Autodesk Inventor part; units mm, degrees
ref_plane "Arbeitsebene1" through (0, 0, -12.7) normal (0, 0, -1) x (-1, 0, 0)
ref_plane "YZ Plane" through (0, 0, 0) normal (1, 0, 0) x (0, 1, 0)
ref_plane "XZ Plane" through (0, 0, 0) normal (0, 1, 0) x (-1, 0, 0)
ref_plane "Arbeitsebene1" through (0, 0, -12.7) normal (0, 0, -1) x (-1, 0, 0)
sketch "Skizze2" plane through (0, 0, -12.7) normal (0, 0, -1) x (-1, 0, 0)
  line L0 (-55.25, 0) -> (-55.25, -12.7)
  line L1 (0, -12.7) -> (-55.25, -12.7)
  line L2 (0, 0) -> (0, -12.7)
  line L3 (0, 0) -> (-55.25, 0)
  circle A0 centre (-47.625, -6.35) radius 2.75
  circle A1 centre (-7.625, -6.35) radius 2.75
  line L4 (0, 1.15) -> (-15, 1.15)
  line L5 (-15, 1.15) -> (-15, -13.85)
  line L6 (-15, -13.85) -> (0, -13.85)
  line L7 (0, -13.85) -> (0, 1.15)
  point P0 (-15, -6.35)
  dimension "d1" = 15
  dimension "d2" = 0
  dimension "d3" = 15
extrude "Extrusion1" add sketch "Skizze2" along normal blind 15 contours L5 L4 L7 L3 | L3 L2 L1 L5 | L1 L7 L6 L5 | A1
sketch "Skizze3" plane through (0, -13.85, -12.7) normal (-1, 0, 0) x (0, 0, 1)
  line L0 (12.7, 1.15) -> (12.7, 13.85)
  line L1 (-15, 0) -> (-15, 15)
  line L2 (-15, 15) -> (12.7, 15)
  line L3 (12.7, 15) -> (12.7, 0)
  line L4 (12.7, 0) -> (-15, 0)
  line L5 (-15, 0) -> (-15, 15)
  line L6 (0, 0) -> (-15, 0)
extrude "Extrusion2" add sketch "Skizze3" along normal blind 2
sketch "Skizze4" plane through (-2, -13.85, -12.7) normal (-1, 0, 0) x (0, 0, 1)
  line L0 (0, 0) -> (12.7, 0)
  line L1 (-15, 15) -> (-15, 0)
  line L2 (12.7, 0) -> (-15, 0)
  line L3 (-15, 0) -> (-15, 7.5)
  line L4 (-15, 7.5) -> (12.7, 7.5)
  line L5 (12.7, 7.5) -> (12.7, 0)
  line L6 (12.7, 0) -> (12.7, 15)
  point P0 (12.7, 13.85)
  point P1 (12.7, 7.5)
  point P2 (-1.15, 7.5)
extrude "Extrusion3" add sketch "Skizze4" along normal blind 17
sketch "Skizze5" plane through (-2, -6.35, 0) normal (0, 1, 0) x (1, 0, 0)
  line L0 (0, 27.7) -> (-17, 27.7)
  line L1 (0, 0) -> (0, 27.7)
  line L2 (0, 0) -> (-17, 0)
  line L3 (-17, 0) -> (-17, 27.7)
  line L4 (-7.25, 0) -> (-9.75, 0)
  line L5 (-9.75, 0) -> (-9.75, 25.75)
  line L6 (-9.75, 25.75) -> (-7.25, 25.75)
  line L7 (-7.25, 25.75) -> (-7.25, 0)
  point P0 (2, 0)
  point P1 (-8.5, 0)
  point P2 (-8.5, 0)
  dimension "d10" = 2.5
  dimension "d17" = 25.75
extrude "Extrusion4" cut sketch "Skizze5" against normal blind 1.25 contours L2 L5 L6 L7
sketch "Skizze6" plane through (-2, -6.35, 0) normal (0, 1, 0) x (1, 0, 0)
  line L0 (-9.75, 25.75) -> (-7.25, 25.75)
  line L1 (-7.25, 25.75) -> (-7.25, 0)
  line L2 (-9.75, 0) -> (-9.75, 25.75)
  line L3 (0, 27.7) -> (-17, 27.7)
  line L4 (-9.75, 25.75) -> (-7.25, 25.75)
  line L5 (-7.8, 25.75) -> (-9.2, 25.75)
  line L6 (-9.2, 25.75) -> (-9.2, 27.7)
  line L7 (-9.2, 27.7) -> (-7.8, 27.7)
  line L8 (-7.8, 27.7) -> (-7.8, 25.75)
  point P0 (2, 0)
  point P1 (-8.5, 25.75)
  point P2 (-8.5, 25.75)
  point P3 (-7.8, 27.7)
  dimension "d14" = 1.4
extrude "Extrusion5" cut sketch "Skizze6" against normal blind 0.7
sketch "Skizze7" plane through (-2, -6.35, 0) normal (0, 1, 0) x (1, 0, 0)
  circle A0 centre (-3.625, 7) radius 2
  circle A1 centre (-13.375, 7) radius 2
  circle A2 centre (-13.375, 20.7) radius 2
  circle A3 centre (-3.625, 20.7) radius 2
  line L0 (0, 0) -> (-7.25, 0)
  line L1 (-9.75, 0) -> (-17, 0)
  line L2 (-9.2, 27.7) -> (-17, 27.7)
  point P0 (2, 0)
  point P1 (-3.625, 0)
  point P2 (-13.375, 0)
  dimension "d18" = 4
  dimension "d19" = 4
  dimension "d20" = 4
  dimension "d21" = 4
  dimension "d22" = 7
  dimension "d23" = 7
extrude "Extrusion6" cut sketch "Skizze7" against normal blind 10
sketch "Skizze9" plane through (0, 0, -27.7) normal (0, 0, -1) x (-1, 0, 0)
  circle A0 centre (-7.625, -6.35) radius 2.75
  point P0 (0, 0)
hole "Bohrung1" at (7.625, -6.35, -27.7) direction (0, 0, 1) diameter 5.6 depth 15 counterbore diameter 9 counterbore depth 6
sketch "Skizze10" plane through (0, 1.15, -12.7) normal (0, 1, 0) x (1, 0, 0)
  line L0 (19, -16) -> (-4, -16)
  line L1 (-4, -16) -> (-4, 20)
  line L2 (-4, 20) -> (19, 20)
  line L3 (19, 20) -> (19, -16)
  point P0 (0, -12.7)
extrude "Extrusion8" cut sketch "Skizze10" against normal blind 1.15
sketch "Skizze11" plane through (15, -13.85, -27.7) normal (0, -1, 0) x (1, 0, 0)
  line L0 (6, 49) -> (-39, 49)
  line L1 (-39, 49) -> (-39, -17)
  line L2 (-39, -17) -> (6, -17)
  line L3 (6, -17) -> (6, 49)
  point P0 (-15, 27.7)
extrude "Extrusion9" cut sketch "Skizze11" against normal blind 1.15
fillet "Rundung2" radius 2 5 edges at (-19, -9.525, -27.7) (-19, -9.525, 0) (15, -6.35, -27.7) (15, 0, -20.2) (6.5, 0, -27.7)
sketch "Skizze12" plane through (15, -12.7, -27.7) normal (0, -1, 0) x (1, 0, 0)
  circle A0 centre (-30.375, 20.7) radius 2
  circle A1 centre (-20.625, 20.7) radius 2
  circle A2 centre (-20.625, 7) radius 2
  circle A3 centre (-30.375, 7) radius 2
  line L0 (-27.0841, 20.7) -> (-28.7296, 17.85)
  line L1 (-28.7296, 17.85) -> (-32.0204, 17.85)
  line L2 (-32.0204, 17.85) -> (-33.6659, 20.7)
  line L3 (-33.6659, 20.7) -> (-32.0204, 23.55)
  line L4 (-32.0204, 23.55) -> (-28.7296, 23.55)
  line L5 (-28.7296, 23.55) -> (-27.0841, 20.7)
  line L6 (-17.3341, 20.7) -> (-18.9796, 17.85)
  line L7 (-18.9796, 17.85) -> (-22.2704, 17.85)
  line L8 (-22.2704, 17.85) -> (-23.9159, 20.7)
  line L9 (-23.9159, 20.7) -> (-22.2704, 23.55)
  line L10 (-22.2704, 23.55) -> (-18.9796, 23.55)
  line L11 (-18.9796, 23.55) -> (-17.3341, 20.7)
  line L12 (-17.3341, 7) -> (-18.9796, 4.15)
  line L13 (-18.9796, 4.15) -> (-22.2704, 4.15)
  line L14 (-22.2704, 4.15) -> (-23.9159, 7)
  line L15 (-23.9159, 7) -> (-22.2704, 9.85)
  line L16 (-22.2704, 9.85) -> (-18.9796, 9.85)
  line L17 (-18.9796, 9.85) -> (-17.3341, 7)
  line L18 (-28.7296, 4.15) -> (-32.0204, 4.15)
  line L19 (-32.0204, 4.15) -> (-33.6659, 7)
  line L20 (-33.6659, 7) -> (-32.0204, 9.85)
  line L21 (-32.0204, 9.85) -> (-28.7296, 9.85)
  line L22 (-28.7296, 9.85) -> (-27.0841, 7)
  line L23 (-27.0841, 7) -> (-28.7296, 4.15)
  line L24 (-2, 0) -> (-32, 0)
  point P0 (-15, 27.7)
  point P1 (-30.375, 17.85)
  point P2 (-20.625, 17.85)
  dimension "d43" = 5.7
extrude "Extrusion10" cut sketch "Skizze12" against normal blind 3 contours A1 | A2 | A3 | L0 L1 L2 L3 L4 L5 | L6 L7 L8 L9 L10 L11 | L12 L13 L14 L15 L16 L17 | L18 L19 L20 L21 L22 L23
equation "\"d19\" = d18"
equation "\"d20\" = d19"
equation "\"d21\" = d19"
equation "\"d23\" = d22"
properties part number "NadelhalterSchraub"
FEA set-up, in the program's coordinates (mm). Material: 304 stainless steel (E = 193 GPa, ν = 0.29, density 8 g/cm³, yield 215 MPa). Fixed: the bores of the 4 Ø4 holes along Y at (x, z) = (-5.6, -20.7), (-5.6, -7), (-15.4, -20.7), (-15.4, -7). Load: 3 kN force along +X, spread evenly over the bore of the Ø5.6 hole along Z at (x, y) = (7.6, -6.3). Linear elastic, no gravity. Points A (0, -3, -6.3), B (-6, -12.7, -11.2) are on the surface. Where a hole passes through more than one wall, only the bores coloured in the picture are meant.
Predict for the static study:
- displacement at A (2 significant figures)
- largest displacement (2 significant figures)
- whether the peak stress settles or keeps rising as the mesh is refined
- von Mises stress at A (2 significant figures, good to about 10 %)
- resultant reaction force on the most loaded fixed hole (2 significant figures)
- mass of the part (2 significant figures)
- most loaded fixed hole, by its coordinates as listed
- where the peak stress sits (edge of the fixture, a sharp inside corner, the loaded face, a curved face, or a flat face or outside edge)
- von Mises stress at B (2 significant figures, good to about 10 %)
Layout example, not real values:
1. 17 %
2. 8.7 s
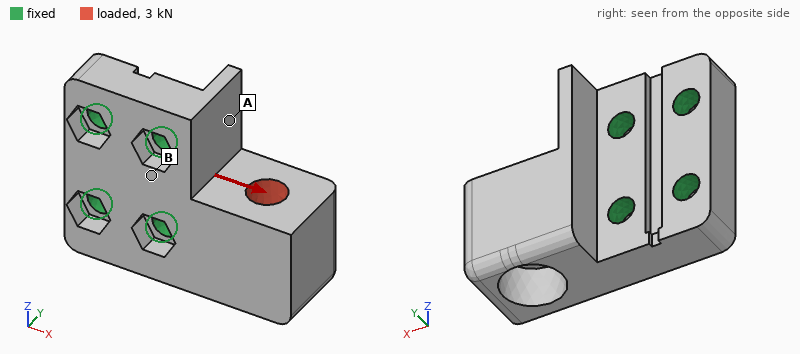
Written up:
1. 3.6 µm
2. 21 µm
3. keeps rising
4. 37 MPa
5. 2.2 kN
6. 42 g
7. (-5.6, -20.7)
8. edge of the fixture
9. 19 MPa
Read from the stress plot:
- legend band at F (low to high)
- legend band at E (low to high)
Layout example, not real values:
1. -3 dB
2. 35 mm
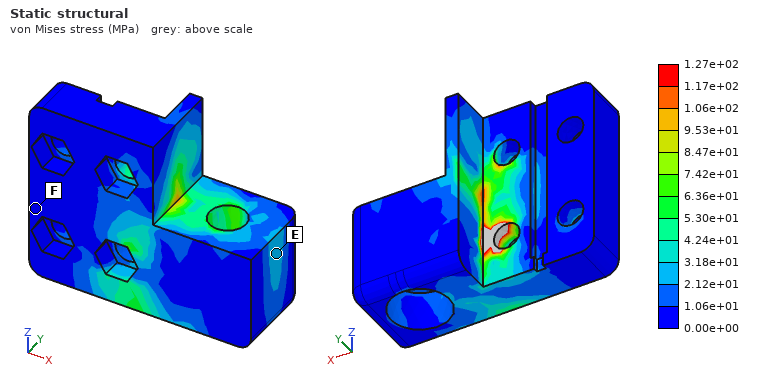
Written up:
1. 0.00e+00 to 1.06e+01 MPa
2. 2.12e+01 to 3.18e+01 MPa
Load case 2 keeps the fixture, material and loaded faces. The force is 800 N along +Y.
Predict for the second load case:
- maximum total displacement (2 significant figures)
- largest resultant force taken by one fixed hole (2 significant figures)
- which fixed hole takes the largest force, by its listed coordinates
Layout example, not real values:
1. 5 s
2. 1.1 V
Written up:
1. 25 µm
2. 1.1 kN
3. (-5.6, -20.7)
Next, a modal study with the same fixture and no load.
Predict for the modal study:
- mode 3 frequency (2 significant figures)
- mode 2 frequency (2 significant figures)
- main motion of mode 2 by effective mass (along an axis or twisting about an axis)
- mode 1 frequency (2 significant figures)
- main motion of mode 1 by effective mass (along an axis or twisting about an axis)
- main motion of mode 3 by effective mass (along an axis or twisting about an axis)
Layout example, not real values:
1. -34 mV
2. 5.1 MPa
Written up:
1. 25 kHz
2. 16 kHz
3. along Z
4. 7800 Hz
5. along Y
6. twisting about X
